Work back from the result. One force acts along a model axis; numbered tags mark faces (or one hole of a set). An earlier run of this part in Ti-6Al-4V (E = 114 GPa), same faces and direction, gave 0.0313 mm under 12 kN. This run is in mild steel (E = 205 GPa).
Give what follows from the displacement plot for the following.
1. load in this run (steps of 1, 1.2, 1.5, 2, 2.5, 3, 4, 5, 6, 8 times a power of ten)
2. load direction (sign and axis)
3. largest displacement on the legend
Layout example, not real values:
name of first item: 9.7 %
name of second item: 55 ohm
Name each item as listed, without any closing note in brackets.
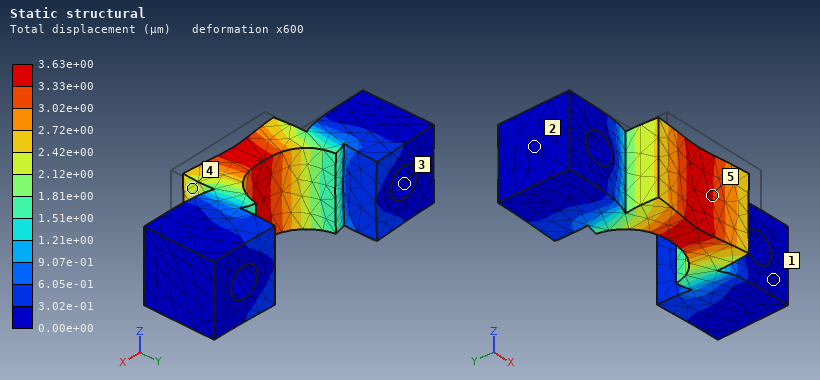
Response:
load in this run: 2.5 kN
load direction: +Y
largest displacement on the legend: 3.63e+00 µm
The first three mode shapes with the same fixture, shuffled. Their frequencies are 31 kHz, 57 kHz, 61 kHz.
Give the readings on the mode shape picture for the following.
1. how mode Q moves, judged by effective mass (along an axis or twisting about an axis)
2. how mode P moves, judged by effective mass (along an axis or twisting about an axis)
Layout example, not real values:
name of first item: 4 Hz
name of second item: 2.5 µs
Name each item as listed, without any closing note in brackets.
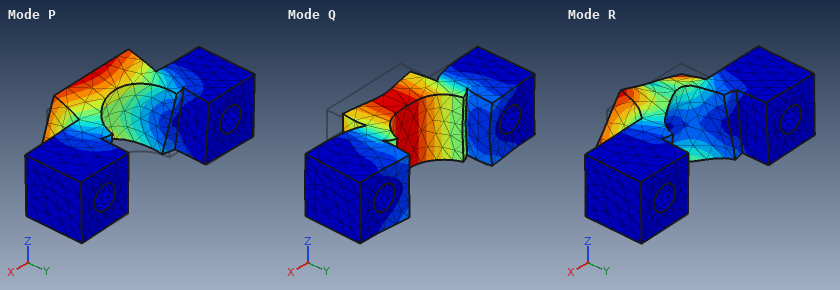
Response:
how mode Q moves, judged by effective mass: along Y
how mode P moves, judged by effective mass: along Z
